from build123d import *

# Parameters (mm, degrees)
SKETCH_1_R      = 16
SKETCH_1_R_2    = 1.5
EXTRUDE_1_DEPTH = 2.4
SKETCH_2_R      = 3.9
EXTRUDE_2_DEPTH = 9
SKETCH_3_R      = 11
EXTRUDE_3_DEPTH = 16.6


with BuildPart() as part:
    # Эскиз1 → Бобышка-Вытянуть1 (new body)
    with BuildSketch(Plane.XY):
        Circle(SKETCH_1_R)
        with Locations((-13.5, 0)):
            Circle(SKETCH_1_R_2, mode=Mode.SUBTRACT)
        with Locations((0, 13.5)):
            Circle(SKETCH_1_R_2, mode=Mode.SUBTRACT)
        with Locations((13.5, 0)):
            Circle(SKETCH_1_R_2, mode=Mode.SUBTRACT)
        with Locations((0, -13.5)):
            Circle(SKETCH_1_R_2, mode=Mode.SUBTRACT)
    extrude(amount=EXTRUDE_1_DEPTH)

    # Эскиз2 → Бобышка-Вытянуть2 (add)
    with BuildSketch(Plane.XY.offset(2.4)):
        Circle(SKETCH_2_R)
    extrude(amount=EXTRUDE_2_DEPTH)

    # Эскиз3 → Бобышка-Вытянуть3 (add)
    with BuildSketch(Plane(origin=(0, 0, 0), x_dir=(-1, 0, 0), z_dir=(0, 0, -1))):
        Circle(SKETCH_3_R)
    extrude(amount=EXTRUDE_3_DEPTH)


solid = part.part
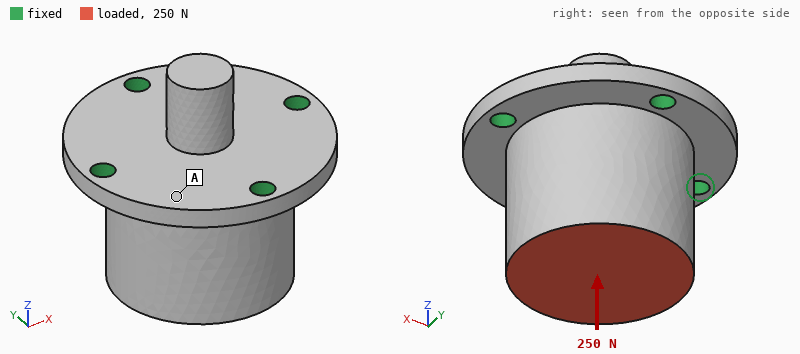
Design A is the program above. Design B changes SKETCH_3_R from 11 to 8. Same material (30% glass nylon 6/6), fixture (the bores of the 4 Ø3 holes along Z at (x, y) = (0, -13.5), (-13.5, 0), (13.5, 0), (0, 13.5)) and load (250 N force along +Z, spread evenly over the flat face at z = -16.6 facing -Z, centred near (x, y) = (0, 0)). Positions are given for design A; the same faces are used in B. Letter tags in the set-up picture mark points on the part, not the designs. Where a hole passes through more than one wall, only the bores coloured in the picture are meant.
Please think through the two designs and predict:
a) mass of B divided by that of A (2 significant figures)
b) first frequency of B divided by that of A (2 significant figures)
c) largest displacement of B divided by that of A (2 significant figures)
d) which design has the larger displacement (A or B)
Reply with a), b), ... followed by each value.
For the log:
a) 0.65
b) 0.75
c) 2.9
d) B
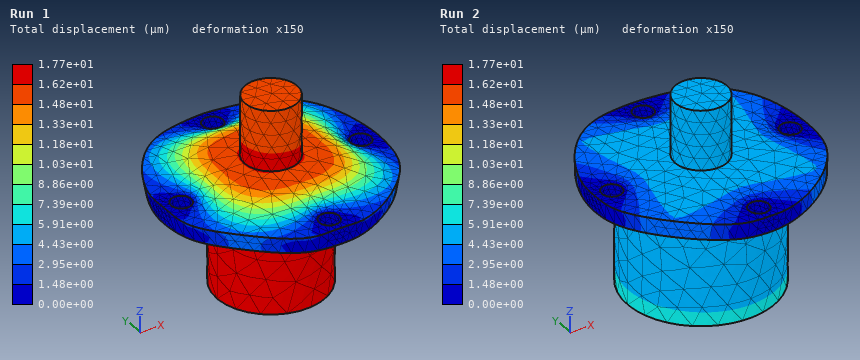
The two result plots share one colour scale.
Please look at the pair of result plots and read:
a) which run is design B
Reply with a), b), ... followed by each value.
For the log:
a) Run 1
